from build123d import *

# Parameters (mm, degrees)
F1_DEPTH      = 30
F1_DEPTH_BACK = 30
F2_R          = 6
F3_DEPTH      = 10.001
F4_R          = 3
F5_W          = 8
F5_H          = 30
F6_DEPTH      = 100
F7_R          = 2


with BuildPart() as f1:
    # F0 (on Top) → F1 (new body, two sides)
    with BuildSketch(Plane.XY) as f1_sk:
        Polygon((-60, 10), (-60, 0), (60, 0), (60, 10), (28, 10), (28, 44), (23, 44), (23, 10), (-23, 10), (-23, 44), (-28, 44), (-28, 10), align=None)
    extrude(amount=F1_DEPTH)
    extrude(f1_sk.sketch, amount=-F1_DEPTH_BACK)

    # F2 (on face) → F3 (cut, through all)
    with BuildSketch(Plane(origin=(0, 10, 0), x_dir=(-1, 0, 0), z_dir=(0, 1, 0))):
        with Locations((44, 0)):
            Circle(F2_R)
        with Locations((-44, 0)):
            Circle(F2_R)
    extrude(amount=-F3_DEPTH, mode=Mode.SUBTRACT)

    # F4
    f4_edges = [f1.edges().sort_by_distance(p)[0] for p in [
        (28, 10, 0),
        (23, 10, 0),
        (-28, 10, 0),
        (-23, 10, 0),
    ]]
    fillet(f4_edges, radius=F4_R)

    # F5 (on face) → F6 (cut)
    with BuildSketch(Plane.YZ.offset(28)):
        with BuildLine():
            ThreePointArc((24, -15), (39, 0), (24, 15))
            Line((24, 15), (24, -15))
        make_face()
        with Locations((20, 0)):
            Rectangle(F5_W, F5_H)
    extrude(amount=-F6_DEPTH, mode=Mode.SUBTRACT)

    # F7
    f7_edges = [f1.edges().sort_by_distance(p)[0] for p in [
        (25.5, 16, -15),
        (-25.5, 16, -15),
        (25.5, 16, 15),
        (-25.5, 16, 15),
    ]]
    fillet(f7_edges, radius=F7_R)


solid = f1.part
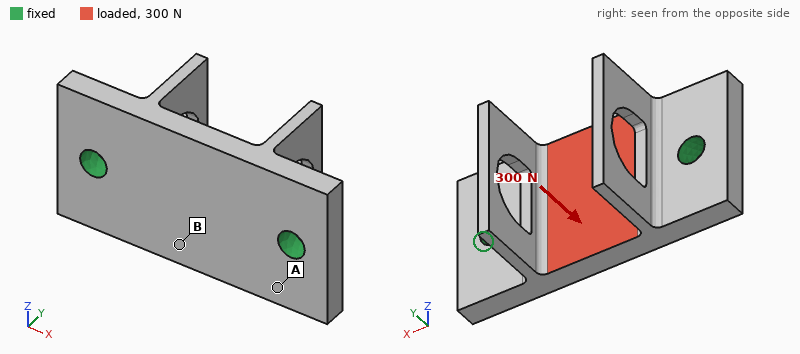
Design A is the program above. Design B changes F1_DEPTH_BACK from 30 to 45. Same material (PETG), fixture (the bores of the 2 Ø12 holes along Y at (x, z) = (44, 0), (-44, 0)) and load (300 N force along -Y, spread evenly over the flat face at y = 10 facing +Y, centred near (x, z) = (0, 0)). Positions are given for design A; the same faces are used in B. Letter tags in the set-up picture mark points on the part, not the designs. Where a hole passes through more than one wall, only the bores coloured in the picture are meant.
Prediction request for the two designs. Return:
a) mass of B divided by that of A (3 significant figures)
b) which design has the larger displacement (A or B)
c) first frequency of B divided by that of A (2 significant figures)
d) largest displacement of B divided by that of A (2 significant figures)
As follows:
1.27
B
1.0
1.3
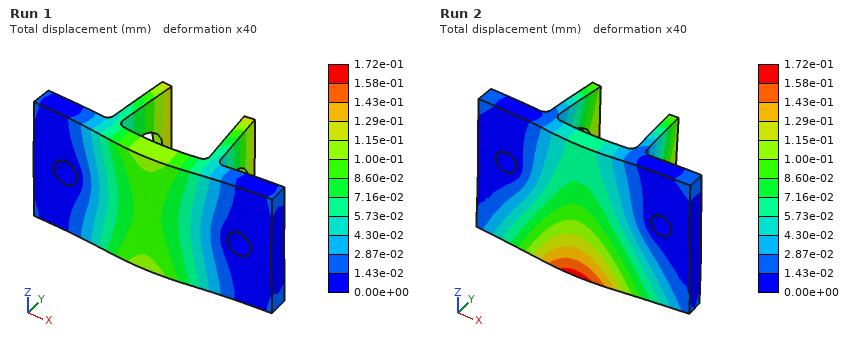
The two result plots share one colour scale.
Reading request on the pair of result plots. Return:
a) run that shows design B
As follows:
Run 2
